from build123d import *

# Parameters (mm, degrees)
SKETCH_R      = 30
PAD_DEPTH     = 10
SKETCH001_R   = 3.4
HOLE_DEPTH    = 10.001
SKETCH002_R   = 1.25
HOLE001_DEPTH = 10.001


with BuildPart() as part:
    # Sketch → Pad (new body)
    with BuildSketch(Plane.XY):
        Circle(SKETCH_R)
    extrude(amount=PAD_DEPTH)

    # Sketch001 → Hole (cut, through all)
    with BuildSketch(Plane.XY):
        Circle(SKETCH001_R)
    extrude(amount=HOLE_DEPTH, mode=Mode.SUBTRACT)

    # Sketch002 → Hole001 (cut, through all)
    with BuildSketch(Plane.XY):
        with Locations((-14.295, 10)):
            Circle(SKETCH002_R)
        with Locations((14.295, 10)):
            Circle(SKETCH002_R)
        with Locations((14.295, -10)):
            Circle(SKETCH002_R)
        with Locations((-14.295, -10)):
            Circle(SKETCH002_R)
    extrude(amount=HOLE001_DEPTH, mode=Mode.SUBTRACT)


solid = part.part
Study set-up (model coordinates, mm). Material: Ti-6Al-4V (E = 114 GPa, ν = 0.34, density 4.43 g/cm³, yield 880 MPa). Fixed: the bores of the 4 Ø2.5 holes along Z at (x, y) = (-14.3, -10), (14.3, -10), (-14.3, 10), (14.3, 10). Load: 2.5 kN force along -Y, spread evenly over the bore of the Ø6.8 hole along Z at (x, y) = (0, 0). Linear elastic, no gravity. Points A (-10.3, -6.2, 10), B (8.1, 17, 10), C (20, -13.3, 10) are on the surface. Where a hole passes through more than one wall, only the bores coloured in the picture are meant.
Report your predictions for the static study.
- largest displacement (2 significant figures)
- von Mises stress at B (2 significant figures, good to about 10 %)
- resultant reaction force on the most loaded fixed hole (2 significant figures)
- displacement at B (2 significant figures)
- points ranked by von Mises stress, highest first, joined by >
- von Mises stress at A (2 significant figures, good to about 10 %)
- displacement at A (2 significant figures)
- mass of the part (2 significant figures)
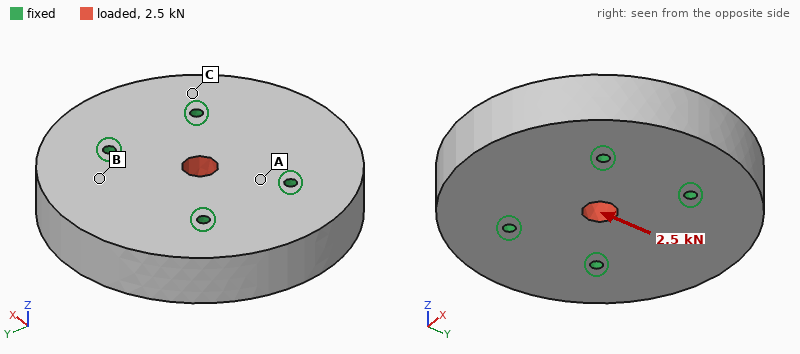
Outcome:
1.4 µm
3.4 MPa
650 N
0.49 µm
A > B > C
6.6 MPa
0.38 µm
120 g
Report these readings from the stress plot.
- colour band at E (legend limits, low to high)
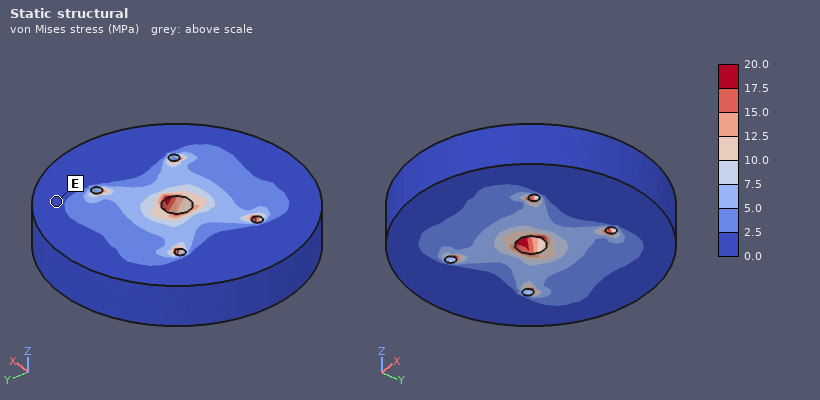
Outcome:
0.0 to 2.5 MPa
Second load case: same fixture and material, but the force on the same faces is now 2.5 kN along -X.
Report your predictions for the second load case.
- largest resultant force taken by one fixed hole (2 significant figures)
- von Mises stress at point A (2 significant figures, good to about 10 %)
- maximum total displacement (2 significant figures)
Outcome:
650 N
7.0 MPa
1.1 µm
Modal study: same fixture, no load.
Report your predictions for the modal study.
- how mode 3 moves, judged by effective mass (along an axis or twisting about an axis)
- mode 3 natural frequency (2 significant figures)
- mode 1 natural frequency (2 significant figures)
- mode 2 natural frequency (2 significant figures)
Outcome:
twisting about Y
25 kHz
16 kHz
16 kHz
